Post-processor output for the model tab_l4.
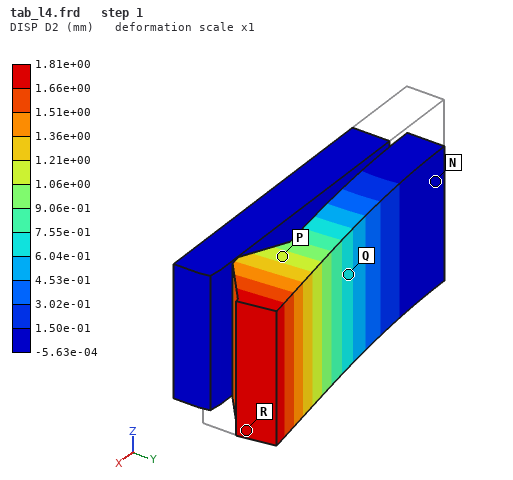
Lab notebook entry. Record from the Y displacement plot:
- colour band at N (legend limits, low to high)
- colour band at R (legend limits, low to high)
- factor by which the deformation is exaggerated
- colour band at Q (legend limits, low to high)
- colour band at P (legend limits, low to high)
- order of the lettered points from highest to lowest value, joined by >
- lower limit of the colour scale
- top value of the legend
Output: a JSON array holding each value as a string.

["-5.63e-04 to 1.50e-01 mm", "1.66e+00 to 1.81e+00 mm", "1", "6.04e-01 to 7.55e-01 mm", "1.06e+00 to 1.21e+00 mm", "R > P > Q > N", "-5.63e-04 mm", "1.81e+00 mm"]
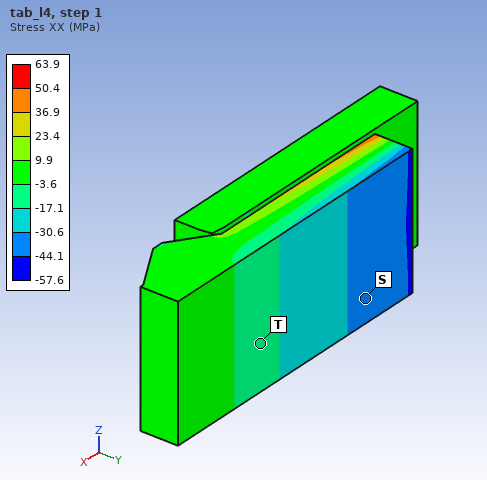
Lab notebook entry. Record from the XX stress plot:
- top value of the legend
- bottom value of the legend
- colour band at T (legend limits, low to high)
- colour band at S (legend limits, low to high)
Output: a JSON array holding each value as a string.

["63.9 MPa", "-57.6 MPa", "-17.1 to -3.6 MPa", "-44.1 to -30.6 MPa"]
